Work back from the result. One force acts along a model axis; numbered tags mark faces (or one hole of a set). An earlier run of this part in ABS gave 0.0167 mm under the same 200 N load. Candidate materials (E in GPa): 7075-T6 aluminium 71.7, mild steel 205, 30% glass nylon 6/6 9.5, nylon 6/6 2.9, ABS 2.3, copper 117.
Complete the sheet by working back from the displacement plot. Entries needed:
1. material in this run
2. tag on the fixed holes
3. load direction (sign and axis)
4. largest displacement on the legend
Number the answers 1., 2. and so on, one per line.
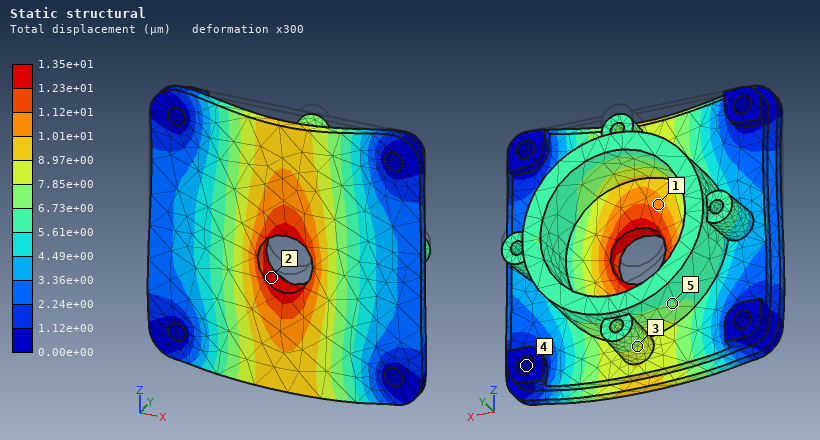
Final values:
1. nylon 6/6
2. 4
3. -Z
4. 1.35e+01 µm
